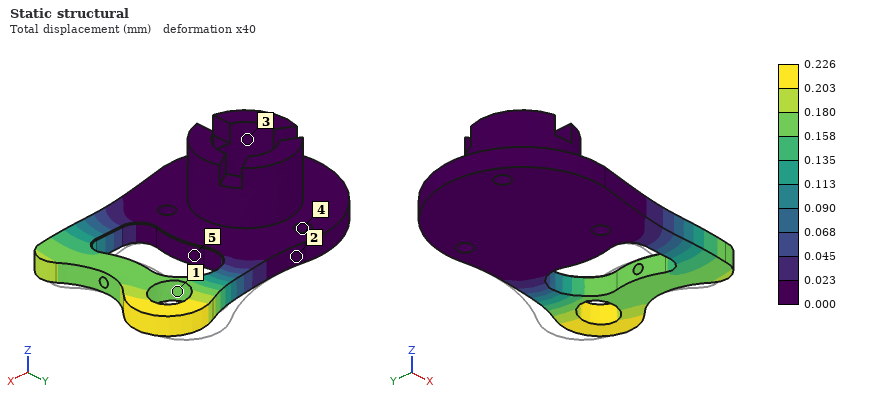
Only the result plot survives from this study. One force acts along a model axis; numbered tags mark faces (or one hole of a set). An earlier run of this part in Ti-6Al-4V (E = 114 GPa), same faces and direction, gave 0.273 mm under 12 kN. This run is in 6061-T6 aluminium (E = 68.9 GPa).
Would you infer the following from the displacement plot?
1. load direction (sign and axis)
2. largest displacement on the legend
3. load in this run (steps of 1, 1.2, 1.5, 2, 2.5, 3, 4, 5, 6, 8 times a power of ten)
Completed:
-Y
0.226 mm
6 kN
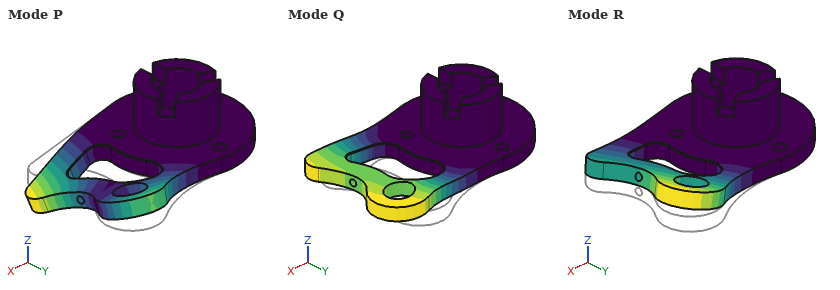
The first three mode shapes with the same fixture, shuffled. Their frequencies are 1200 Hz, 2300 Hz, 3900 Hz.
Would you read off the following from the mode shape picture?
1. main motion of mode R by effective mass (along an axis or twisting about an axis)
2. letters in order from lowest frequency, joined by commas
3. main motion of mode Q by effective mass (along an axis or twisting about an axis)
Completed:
along Z
R, P, Q
along Y
